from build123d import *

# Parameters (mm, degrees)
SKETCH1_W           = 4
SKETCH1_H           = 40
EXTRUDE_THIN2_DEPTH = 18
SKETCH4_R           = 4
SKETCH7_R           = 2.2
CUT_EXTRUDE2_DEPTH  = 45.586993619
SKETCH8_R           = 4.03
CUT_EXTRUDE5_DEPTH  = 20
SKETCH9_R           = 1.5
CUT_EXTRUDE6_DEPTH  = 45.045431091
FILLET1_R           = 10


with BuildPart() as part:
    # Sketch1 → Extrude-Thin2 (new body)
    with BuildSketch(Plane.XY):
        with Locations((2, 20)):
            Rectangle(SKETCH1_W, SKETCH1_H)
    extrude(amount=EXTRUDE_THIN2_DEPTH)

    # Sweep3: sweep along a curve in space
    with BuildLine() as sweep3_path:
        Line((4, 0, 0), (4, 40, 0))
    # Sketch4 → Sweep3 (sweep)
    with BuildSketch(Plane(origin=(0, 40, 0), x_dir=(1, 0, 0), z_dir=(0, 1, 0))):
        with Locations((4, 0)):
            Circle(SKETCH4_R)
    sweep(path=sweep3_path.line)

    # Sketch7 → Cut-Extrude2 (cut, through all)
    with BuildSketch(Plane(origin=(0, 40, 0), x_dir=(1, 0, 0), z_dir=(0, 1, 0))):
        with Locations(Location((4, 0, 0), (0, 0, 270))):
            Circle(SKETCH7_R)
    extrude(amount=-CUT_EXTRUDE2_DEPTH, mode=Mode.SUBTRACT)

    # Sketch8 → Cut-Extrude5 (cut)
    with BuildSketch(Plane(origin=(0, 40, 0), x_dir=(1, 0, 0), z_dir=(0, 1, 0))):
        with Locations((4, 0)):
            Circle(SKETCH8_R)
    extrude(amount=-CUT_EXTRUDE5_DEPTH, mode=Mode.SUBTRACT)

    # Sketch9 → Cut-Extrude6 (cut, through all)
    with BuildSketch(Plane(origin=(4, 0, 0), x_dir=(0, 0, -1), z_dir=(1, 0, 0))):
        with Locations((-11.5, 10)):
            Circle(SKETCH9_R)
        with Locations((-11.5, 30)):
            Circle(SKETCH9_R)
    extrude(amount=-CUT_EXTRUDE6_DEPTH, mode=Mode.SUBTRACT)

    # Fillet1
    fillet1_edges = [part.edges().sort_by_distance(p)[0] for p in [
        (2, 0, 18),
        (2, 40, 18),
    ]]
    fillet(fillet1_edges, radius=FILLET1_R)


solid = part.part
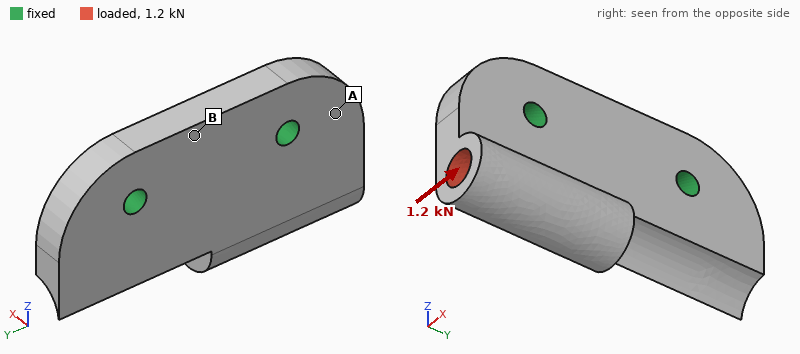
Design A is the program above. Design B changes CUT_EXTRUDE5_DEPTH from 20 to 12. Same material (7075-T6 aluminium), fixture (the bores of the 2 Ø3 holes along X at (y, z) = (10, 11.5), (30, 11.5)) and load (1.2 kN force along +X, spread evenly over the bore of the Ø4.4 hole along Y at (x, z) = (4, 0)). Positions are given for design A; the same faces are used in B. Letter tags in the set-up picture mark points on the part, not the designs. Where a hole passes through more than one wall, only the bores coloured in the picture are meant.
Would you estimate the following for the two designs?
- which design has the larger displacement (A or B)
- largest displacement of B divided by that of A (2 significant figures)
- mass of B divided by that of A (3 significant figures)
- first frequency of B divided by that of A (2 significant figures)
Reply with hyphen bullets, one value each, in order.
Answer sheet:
- A
- 0.75
- 1.10
- 0.98
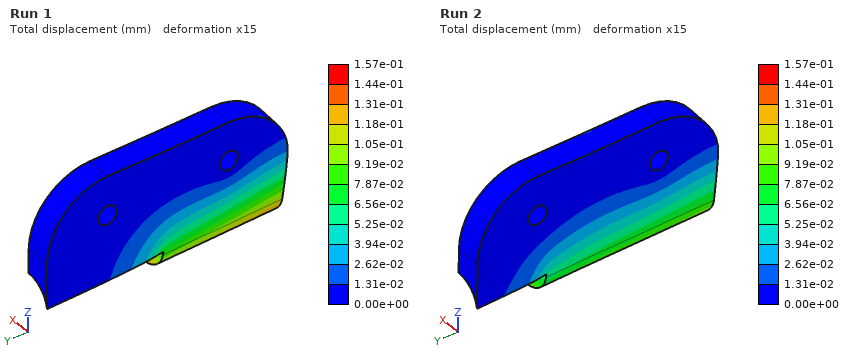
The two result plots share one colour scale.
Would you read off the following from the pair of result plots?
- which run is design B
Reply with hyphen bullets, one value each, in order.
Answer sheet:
- Run 2
